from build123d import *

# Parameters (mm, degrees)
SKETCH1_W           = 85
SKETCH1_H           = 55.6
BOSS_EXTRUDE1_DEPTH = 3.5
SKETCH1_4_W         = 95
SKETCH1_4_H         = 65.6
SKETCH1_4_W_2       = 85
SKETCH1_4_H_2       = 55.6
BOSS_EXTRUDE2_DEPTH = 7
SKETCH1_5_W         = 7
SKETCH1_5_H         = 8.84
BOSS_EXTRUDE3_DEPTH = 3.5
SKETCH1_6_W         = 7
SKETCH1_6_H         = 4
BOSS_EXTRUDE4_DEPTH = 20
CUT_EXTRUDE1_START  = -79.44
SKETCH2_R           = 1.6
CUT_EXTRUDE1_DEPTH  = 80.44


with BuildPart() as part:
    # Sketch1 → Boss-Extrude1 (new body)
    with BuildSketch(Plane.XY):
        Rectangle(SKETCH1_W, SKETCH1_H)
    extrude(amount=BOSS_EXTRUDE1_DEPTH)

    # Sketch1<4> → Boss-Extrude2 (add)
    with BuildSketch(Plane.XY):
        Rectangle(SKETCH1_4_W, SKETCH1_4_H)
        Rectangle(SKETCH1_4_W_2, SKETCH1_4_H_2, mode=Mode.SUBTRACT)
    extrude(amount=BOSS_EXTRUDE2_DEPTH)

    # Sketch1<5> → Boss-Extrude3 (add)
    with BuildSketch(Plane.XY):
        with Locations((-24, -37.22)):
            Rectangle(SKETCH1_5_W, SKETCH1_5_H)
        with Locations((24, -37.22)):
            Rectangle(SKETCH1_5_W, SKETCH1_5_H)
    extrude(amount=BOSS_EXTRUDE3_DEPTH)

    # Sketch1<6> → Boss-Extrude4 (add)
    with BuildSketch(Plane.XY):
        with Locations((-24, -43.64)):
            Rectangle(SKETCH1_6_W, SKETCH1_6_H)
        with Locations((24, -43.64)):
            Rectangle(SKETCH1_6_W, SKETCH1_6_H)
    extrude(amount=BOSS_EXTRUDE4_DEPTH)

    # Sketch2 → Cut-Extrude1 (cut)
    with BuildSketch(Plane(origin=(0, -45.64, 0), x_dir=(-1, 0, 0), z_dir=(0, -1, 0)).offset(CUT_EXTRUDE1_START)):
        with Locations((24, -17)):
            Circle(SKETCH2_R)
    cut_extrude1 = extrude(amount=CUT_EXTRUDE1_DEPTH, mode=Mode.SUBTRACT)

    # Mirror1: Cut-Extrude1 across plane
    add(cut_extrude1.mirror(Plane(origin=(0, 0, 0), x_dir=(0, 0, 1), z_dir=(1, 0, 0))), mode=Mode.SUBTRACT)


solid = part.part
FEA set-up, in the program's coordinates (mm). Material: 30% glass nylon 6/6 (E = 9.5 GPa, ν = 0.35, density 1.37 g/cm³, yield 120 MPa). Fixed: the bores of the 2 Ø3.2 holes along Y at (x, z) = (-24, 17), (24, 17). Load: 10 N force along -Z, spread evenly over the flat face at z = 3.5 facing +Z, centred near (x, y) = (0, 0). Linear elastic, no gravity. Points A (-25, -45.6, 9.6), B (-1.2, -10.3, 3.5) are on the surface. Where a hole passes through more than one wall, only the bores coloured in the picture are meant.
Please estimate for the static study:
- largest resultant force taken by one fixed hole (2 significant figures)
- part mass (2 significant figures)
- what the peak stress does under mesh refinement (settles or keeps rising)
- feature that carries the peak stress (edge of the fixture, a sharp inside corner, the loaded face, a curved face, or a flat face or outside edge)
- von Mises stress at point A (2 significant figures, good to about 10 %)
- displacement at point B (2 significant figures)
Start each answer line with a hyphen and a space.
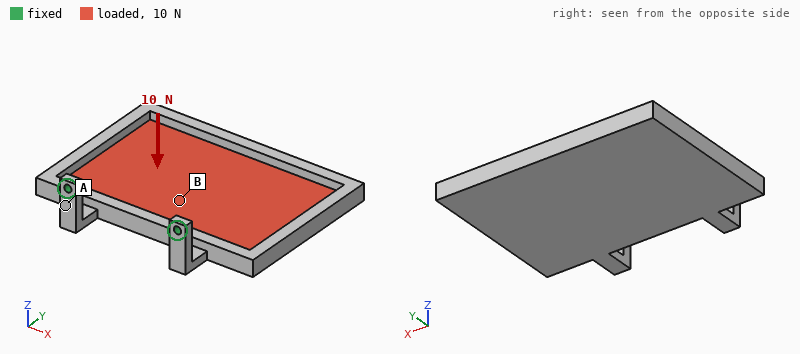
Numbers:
- 5.0 N
- 39 g
- keeps rising
- edge of the fixture
- 12 MPa
- 0.54 mm
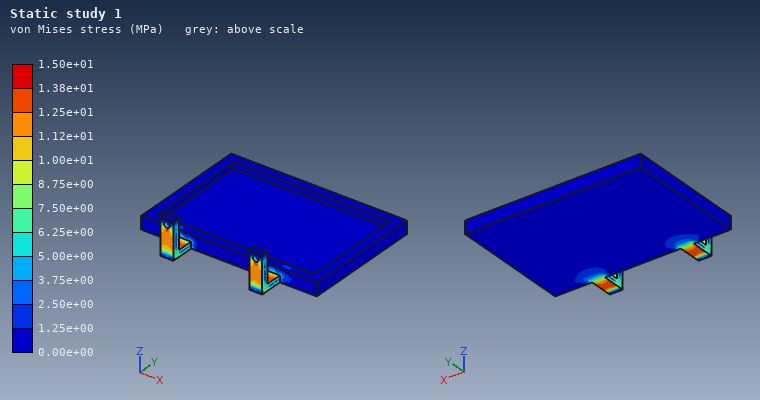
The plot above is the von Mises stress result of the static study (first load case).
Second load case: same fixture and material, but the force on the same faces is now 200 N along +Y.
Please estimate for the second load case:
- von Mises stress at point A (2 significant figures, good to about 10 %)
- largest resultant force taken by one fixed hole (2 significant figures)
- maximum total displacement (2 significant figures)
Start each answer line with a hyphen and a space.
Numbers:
- 32 MPa
- 100 N
- 1.1 mm
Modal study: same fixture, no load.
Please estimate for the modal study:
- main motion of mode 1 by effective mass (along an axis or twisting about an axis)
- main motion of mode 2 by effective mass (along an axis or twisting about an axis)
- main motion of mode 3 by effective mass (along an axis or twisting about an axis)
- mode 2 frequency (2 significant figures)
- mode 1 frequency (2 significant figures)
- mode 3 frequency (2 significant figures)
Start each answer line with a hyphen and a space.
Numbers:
- along Z
- along X
- along X
- 300 Hz
- 85 Hz
- 430 Hz
